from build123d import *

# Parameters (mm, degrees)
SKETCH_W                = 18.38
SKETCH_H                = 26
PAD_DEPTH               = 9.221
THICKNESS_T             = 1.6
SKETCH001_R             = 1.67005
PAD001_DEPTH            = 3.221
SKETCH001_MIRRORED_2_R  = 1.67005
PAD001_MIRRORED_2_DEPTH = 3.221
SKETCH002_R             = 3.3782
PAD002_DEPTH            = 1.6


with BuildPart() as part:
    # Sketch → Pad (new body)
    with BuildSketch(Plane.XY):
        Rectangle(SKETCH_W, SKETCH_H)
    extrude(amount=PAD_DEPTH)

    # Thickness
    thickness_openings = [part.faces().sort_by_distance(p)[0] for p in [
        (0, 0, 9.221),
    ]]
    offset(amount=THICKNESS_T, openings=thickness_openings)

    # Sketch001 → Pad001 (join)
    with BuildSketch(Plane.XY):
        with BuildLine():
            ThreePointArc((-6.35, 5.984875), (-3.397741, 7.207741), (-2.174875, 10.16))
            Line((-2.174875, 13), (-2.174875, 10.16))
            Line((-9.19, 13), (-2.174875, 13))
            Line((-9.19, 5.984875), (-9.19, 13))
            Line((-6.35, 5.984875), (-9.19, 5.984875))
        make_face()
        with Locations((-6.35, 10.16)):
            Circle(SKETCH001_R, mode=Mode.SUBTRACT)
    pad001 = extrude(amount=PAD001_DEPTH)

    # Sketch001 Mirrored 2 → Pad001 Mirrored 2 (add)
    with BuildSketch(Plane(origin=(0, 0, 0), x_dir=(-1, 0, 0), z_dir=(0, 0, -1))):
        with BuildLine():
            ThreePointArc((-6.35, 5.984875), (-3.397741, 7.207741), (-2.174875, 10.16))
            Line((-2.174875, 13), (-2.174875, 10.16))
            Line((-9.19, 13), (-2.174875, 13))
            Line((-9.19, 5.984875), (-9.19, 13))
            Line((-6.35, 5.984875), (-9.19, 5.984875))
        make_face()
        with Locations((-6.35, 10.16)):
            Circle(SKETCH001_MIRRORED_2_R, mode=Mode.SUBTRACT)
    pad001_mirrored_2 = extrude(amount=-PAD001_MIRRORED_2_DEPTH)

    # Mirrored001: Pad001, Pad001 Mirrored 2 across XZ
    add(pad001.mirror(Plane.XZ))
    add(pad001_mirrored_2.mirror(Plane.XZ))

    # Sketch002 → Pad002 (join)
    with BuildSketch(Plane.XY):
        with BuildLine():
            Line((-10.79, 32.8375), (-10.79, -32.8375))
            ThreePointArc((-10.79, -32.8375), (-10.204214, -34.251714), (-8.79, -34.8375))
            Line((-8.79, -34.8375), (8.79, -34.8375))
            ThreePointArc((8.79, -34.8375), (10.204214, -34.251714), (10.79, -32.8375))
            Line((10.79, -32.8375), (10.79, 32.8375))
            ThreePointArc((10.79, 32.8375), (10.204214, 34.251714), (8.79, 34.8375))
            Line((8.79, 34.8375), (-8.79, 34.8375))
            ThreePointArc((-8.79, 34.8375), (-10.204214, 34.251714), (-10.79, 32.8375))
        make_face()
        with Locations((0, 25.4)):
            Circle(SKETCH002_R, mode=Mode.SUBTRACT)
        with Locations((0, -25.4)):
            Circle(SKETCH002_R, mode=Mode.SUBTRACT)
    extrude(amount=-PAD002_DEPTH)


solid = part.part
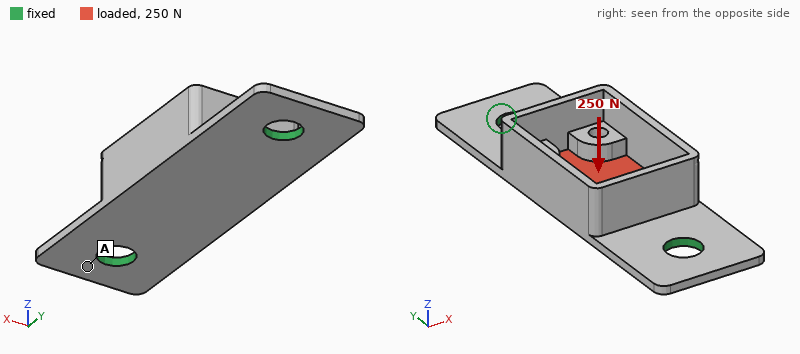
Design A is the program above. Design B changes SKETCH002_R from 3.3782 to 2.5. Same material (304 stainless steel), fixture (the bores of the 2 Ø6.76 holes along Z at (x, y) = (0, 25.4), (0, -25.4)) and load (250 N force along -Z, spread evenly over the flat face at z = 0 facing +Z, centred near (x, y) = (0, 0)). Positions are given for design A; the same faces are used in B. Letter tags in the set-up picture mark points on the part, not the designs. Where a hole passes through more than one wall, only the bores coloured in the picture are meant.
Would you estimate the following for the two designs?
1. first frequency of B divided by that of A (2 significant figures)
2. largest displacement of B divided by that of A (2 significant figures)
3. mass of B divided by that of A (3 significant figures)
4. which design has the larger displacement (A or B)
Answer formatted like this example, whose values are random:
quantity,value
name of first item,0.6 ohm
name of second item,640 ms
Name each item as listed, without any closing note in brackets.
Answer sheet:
quantity,value
first frequency of B divided by that of A,0.89
largest displacement of B divided by that of A,1.2
mass of B divided by that of A,1.01
which design has the larger displacement,B
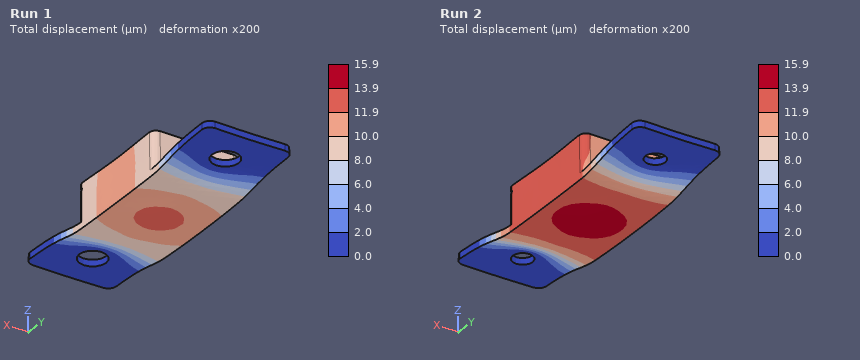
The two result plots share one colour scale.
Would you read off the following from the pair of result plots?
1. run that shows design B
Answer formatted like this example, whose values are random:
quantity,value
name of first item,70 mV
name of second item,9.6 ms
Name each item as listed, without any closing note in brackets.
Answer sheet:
quantity,value
run that shows design B,Run 2
